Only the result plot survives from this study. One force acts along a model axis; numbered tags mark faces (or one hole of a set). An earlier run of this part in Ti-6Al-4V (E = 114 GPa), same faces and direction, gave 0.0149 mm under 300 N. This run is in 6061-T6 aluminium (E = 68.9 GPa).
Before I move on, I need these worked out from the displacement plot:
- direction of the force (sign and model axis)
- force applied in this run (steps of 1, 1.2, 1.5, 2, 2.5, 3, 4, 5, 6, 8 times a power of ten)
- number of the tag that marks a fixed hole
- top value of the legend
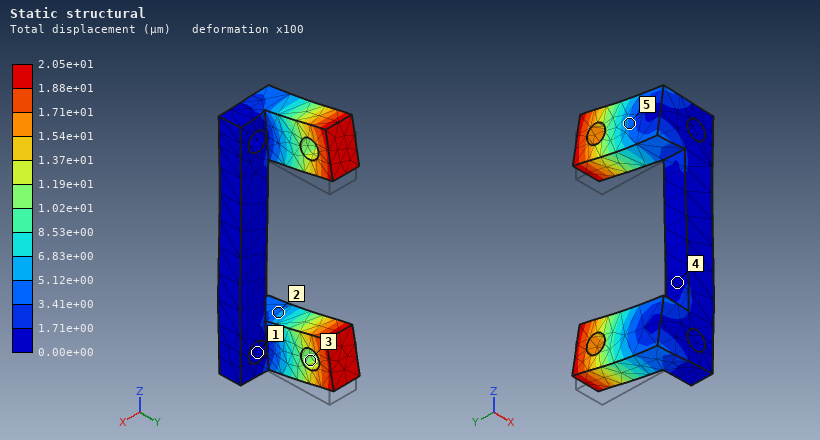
+Z
250 N
1
2.05e+01 µm
